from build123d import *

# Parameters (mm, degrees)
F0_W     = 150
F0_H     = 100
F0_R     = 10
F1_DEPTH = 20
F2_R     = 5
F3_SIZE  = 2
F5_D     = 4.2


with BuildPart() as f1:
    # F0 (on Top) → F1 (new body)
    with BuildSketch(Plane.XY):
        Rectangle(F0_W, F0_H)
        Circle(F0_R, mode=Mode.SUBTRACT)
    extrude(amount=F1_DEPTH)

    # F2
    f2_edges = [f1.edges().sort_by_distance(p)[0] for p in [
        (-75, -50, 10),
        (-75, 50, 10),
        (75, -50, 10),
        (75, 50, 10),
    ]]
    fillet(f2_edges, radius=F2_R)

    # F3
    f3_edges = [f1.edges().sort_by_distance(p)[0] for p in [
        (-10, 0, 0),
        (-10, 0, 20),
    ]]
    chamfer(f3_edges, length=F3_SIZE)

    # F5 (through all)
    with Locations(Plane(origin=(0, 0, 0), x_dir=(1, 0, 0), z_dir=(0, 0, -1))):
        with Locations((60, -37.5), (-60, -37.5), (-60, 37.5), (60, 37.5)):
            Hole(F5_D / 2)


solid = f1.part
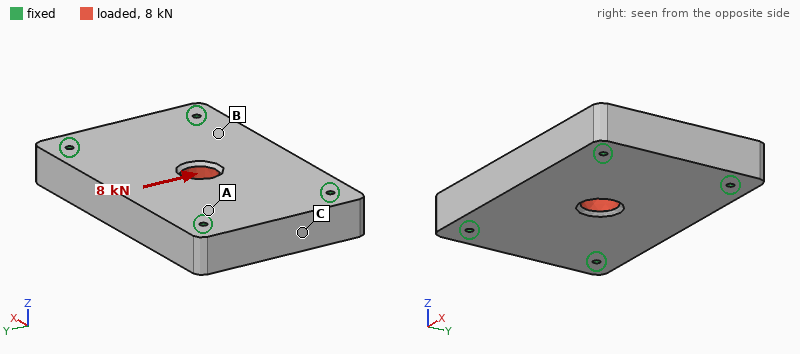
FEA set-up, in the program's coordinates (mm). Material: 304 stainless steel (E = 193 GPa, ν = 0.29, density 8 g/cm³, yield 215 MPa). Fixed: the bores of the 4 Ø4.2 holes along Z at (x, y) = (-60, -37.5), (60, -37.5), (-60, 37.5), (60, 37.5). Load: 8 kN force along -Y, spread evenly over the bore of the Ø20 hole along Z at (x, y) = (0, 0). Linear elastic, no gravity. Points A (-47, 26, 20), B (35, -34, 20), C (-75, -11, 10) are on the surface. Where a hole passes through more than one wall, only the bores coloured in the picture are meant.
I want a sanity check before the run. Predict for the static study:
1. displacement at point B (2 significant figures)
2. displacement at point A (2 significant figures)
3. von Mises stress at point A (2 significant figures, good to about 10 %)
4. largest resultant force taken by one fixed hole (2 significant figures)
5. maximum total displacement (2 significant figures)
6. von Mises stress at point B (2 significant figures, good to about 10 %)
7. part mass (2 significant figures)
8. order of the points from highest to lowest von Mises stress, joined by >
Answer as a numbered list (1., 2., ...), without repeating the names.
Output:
1. 1.2 µm
2. 0.68 µm
3. 4.9 MPa
4. 2.5 kN
5. 2.6 µm
6. 3.3 MPa
7. 2.3 kg
8. A > B > C
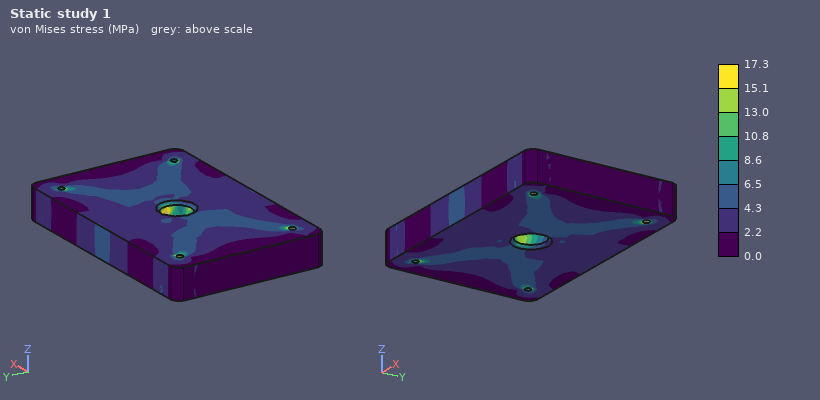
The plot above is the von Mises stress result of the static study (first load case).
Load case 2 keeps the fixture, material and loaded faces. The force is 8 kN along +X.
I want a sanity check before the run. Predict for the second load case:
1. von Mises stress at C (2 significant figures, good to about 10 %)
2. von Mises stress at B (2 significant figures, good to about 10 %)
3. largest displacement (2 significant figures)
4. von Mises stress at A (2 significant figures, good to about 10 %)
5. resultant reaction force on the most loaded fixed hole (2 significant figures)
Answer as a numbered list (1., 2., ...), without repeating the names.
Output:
1. 2.2 MPa
2. 2.8 MPa
3. 1.6 µm
4. 3.6 MPa
5. 2.1 kN
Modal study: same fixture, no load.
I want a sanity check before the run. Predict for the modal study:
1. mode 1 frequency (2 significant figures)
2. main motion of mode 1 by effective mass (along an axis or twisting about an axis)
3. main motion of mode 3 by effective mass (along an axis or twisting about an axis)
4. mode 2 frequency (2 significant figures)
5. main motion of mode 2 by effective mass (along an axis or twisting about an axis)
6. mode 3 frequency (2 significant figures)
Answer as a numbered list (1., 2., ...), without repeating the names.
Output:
1. 4500 Hz
2. along Z
3. along Y
4. 6700 Hz
5. twisting about X
6. 9900 Hz
